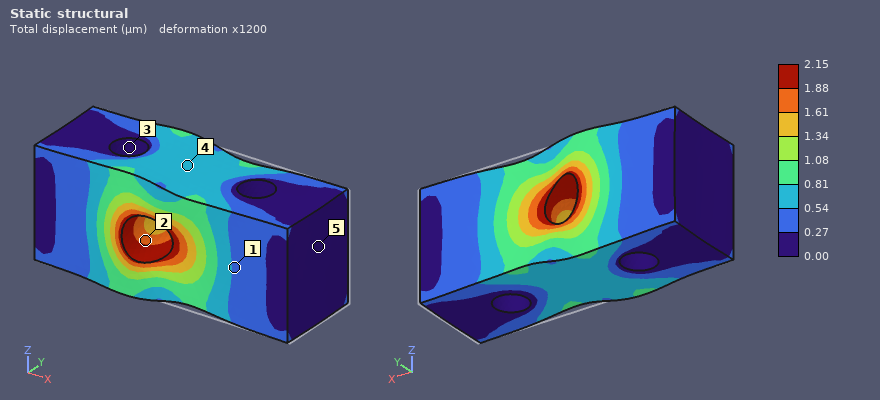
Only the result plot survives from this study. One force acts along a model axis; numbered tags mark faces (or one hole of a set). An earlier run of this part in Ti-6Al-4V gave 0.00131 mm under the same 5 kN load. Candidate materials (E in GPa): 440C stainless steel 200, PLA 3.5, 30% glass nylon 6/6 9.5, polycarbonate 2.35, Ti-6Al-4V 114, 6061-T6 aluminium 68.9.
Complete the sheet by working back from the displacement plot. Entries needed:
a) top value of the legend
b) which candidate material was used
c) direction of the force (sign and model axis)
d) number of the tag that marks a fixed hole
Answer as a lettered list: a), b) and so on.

a) 2.15 µm
b) 6061-T6 aluminium
c) -X
d) 3
